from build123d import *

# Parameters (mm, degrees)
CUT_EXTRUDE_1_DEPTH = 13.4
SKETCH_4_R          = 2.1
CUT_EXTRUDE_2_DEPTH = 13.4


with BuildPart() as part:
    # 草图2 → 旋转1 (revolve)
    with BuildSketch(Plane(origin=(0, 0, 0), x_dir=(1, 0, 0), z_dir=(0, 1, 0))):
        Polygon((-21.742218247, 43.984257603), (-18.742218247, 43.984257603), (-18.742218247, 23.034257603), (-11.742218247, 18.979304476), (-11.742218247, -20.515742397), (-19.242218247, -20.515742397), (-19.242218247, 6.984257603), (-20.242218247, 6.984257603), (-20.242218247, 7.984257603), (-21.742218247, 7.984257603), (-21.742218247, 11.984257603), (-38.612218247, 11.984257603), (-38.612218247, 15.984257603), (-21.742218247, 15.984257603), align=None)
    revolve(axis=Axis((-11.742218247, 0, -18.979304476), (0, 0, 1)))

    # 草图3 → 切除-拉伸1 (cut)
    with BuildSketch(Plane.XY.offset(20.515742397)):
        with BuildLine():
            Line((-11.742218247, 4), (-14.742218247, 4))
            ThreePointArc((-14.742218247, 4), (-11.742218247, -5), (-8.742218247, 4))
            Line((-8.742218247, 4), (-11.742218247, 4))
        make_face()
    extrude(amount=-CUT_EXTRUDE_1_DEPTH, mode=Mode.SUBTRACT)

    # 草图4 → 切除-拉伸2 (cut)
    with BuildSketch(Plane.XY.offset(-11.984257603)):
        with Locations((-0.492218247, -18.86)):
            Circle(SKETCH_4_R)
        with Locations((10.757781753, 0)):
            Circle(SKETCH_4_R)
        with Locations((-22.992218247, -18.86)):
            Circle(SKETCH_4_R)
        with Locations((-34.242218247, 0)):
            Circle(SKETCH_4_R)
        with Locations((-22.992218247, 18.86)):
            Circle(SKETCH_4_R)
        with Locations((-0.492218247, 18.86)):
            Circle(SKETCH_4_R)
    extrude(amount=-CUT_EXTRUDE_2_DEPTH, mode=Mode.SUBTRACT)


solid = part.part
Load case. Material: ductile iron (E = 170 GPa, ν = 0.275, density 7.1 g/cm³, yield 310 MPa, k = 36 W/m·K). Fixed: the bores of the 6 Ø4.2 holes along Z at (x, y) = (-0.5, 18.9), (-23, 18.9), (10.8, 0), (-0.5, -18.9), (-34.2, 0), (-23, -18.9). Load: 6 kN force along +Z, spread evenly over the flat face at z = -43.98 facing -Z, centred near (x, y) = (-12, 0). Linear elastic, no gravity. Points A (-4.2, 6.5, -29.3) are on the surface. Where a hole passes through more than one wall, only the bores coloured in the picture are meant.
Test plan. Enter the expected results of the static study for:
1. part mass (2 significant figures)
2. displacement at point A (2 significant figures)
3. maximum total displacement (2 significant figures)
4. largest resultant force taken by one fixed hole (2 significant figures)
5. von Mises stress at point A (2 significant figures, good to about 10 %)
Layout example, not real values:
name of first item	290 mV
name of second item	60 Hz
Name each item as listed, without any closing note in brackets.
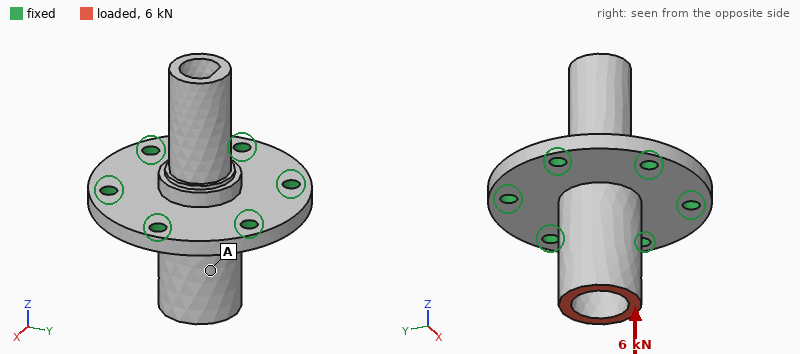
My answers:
part mass	140 g
displacement at point A	20 µm
maximum total displacement	23 µm
largest resultant force taken by one fixed hole	1.0 kN
von Mises stress at point A	37 MPa
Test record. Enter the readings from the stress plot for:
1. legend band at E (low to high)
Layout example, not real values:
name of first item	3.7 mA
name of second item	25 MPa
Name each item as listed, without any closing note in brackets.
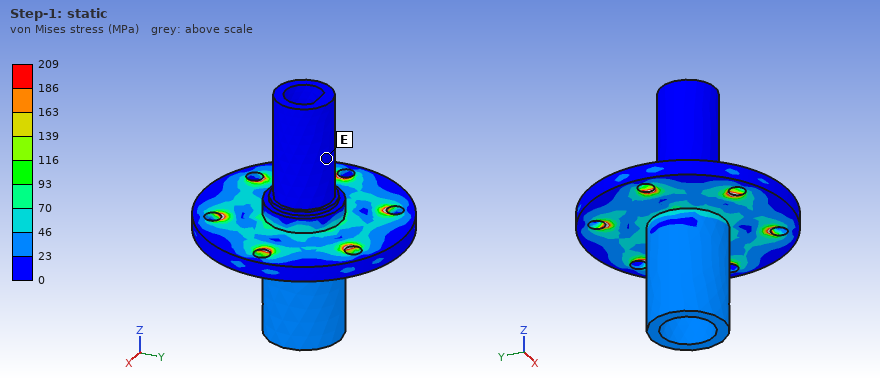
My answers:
legend band at E	0 to 23 MPa
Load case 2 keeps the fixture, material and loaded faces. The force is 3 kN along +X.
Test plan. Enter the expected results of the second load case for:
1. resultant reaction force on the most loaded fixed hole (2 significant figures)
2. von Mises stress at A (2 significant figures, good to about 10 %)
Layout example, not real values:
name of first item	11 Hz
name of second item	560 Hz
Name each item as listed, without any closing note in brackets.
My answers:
resultant reaction force on the most loaded fixed hole	1.8 kN
von Mises stress at A	64 MPa
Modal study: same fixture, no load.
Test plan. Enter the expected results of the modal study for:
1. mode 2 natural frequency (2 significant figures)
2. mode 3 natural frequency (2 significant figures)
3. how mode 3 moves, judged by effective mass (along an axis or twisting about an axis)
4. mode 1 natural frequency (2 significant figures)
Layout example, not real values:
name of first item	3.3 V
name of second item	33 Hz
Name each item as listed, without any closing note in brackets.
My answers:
mode 2 natural frequency	6300 Hz
mode 3 natural frequency	9600 Hz
how mode 3 moves, judged by effective mass	along Z
mode 1 natural frequency	6200 Hz
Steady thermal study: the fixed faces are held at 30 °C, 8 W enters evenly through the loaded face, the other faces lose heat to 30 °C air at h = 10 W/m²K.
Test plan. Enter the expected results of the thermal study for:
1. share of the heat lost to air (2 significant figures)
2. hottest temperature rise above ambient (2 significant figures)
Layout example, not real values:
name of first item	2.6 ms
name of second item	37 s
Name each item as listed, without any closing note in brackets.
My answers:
share of the heat lost to air	12 %
hottest temperature rise above ambient	42 K
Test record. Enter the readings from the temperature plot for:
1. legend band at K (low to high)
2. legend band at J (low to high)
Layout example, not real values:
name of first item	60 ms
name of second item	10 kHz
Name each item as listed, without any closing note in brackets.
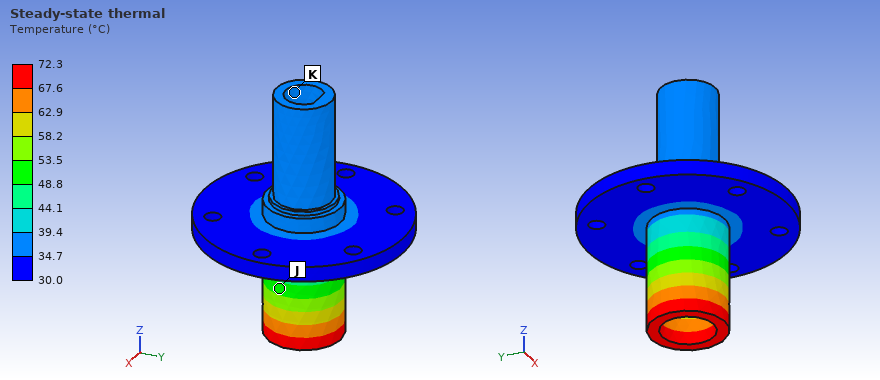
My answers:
legend band at K	34.7 to 39.4 °C
legend band at J	48.8 to 53.5 °C
